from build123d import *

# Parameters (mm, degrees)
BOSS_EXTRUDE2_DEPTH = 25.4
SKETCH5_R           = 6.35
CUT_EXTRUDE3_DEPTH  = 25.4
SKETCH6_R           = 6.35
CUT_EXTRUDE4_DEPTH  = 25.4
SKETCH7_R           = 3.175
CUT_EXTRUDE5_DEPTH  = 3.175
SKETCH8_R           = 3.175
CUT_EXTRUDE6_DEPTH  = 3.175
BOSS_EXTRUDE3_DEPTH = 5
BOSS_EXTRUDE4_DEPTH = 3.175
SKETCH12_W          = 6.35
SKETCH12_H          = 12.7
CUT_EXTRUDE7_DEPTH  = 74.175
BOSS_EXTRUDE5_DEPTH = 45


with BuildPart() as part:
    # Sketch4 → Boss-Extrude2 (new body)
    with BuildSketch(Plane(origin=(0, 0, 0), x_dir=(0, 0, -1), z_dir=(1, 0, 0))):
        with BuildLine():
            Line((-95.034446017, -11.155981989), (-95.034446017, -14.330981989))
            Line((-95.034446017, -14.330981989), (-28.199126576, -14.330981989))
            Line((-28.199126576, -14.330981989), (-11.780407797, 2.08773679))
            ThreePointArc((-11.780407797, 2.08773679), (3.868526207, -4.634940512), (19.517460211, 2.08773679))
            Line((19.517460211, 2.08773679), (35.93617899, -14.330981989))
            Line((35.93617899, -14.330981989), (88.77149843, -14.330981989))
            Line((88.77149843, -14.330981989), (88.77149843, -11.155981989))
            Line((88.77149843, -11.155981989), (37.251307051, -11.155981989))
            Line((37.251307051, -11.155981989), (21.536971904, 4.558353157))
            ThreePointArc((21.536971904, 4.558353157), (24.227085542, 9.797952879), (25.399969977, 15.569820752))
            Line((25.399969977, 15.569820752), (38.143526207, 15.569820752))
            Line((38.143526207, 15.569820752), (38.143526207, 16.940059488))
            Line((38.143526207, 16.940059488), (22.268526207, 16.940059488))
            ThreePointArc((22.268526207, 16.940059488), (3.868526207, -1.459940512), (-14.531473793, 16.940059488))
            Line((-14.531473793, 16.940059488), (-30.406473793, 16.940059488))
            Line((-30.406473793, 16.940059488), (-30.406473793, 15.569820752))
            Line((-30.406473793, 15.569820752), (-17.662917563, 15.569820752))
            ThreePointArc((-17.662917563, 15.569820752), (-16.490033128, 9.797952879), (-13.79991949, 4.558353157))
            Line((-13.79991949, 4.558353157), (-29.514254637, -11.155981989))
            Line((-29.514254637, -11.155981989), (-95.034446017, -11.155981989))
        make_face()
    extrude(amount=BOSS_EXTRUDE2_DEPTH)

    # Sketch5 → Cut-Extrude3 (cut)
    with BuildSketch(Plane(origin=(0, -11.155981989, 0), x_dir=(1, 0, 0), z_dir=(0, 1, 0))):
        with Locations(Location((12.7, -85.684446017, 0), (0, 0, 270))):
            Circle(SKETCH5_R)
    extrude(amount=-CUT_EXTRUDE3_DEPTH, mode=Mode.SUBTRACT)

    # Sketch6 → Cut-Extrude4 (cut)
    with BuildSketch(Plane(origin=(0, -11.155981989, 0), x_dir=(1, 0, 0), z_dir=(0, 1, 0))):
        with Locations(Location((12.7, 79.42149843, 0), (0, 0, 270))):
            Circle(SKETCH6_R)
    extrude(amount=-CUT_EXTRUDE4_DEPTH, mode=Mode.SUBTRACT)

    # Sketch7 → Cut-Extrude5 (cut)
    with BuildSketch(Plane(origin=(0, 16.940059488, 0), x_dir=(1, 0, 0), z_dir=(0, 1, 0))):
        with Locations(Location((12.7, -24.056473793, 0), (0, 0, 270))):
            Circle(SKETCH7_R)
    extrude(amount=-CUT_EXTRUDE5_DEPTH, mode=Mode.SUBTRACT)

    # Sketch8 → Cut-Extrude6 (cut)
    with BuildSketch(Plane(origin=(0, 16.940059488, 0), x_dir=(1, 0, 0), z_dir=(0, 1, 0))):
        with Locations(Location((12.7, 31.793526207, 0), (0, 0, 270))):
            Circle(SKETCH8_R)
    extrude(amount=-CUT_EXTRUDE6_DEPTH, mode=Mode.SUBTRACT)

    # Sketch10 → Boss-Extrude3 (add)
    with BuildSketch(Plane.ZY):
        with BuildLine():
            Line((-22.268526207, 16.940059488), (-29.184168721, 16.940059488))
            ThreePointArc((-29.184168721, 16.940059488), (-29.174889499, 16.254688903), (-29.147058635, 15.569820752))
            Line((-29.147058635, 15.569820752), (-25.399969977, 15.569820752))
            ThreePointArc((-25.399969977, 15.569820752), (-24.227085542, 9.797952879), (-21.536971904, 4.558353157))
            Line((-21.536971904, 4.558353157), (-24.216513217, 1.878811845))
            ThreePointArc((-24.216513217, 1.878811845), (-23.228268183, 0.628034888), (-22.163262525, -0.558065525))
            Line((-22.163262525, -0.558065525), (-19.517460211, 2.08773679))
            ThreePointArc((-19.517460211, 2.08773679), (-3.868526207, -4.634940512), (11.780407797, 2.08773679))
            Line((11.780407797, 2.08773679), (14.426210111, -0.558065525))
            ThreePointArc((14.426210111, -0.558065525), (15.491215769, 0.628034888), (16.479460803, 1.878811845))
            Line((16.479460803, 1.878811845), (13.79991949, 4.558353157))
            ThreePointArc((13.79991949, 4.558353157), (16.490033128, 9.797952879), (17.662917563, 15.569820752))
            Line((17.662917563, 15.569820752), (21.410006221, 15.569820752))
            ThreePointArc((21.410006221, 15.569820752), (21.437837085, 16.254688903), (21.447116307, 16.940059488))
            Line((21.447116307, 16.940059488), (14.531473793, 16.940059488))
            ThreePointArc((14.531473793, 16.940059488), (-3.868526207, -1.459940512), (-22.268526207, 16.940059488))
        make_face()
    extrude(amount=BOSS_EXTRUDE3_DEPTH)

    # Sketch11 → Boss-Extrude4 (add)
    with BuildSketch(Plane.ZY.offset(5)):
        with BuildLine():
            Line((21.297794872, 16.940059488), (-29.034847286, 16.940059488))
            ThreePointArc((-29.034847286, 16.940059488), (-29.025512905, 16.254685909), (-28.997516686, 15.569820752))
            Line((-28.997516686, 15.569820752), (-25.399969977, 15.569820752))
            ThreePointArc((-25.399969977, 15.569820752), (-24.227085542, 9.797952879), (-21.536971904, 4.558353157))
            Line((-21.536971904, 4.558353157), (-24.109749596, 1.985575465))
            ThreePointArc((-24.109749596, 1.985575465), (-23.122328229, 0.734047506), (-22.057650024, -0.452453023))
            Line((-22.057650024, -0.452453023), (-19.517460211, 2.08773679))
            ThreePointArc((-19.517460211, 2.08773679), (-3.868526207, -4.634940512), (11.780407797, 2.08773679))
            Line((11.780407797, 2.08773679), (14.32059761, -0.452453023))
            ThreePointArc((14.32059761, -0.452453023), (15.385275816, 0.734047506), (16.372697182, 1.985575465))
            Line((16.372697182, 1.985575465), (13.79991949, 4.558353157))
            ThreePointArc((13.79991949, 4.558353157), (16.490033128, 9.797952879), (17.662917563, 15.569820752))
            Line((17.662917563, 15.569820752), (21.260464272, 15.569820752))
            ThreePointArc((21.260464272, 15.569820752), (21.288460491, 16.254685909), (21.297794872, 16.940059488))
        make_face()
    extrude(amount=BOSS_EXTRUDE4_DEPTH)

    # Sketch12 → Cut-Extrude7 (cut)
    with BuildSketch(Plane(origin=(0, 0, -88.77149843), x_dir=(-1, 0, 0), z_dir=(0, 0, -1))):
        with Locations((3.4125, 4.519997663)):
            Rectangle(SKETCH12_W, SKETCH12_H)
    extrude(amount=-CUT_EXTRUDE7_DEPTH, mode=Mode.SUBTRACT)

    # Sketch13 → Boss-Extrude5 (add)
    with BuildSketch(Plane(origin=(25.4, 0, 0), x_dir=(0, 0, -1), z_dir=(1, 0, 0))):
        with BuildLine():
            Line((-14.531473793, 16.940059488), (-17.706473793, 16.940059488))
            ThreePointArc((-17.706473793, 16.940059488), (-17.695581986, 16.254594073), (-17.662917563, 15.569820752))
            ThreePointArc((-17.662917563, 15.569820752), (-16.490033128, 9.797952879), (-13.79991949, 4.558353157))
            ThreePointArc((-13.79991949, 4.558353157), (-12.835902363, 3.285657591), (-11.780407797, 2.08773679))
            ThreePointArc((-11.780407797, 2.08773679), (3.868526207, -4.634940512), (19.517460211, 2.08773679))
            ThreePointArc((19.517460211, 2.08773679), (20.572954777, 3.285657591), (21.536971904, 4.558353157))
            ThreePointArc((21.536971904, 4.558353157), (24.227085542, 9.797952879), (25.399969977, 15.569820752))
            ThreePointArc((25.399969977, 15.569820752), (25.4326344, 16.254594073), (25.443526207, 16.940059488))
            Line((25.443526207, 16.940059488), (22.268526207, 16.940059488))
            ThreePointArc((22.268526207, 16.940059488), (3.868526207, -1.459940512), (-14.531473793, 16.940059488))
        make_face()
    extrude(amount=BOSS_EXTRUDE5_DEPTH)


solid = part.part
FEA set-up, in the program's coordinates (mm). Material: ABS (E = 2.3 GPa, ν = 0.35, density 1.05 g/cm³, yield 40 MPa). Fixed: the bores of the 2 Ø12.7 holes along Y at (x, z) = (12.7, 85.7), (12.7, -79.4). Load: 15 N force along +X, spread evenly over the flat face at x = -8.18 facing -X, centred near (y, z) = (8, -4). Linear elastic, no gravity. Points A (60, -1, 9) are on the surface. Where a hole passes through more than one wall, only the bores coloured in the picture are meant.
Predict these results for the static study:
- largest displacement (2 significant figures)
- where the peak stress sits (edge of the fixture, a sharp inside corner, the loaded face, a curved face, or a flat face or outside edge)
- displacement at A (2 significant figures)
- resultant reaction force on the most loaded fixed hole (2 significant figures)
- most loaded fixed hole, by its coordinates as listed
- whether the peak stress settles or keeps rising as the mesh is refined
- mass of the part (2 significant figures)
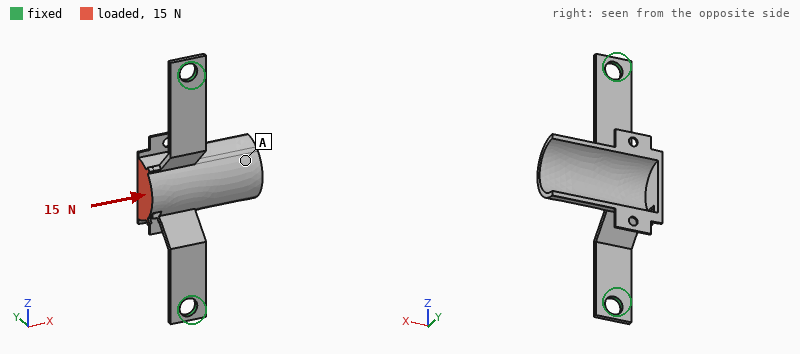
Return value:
1.9 mm
edge of the fixture
1.4 mm
8.8 N
(12.7, -79.4)
keeps rising
32 g
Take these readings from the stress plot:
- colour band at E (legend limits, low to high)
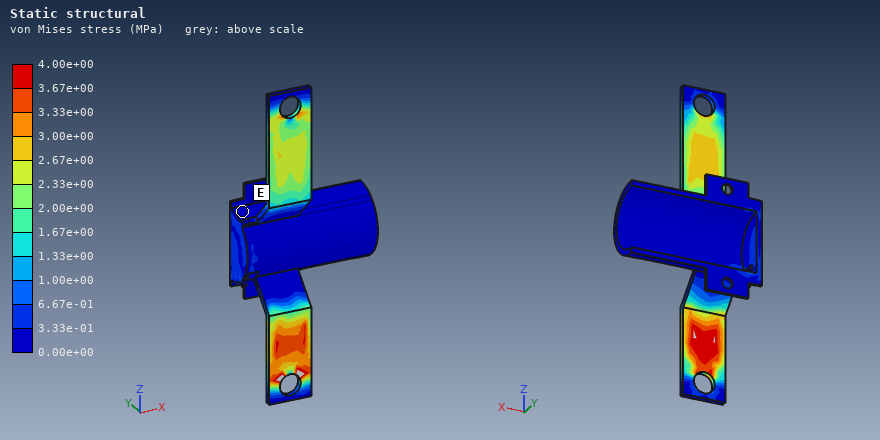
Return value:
0.00e+00 to 3.33e-01 MPa
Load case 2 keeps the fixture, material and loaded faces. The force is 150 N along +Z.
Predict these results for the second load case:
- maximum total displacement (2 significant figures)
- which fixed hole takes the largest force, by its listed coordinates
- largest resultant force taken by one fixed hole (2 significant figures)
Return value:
2.3 mm
(12.7, 85.7)
94 N
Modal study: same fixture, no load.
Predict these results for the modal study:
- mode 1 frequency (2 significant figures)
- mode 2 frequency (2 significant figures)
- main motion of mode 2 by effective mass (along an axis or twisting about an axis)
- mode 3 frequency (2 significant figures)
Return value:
110 Hz
190 Hz
along Y
320 Hz
